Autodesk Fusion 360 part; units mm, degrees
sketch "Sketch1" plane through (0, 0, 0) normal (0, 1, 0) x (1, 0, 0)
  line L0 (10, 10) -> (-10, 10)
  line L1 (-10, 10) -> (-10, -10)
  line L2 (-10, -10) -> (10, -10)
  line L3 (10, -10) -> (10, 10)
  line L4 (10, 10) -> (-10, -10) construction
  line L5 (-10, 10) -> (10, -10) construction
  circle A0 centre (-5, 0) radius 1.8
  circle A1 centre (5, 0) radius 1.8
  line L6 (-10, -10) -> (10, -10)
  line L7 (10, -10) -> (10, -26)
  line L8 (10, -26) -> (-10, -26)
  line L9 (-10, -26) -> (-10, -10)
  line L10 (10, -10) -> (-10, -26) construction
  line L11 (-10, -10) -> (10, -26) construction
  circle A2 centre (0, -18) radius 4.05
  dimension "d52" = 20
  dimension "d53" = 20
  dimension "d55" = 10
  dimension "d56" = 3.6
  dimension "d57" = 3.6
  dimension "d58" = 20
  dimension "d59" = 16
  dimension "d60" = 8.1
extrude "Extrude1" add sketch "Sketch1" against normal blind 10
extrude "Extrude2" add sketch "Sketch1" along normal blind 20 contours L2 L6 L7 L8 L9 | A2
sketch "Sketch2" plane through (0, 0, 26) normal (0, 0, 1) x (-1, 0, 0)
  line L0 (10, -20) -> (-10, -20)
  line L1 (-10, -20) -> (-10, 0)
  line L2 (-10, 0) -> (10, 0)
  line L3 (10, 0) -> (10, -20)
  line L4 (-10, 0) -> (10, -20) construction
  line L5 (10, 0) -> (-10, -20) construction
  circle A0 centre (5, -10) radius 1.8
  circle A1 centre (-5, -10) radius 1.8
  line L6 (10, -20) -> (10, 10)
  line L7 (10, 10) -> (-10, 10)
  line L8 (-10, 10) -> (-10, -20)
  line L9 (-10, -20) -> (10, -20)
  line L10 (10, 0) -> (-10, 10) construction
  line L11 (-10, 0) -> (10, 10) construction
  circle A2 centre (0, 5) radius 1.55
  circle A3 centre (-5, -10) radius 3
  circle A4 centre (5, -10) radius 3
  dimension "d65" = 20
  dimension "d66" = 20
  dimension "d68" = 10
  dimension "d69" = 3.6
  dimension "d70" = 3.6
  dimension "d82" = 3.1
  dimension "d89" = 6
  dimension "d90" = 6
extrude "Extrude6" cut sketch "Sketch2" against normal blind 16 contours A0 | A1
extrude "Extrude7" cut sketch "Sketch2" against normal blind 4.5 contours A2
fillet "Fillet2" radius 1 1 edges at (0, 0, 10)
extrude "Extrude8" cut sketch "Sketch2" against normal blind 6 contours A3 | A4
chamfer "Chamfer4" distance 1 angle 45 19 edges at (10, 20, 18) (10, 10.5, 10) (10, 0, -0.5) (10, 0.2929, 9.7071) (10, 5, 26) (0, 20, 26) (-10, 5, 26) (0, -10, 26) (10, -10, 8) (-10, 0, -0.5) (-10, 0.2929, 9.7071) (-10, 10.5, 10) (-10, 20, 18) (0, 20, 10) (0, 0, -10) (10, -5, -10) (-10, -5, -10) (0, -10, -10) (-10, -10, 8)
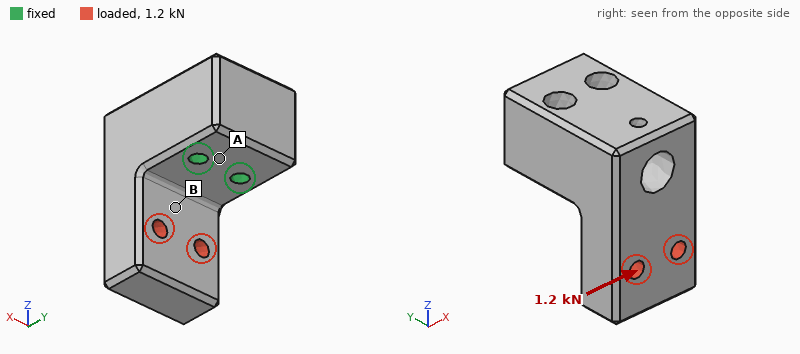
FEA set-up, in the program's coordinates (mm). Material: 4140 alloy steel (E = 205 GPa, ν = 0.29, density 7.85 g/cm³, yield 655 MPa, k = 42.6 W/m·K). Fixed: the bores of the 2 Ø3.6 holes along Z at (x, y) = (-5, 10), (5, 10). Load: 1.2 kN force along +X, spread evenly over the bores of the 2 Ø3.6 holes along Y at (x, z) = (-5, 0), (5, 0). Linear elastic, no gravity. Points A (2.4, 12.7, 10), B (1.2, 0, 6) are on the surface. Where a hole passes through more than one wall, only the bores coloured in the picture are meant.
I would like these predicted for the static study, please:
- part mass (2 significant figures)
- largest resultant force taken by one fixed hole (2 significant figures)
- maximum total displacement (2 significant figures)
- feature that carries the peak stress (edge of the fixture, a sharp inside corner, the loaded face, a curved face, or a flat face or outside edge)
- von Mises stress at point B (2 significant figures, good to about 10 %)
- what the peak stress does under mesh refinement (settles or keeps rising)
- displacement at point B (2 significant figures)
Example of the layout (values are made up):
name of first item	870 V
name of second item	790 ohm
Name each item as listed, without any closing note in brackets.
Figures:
part mass	95 g
largest resultant force taken by one fixed hole	1.8 kN
maximum total displacement	13 µm
feature that carries the peak stress	edge of the fixture
von Mises stress at point B	19 MPa
what the peak stress does under mesh refinement	keeps rising
displacement at point B	5.1 µm
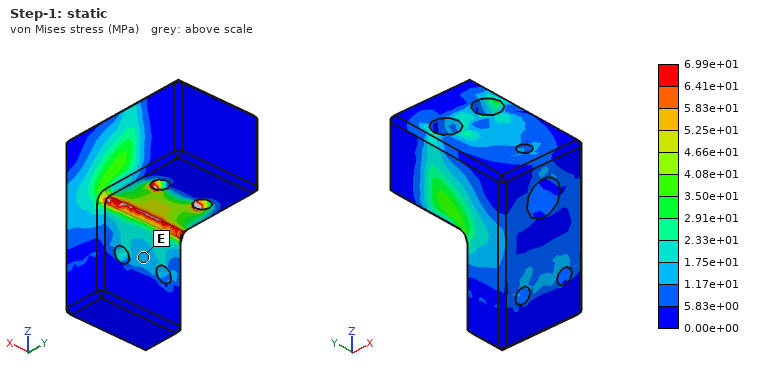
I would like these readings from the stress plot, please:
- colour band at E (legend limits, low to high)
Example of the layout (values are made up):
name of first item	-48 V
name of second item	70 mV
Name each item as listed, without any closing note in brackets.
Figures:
colour band at E	1.17e+01 to 1.75e+01 MPa
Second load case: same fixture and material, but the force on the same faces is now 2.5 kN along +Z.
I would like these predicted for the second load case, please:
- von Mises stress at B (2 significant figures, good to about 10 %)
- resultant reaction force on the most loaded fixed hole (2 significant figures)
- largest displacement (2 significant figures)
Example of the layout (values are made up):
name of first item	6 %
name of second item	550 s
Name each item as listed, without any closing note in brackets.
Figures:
von Mises stress at B	14 MPa
resultant reaction force on the most loaded fixed hole	1.3 kN
largest displacement	17 µm
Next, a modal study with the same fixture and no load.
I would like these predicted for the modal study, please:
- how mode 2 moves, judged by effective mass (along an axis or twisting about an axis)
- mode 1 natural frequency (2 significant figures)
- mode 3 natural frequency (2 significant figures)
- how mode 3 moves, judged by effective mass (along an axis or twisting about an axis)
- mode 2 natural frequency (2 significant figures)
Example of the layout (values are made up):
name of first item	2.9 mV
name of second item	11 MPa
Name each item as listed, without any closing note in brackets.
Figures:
how mode 2 moves, judged by effective mass	along X
mode 1 natural frequency	8000 Hz
mode 3 natural frequency	18 kHz
how mode 3 moves, judged by effective mass	along Z
mode 2 natural frequency	10 kHz
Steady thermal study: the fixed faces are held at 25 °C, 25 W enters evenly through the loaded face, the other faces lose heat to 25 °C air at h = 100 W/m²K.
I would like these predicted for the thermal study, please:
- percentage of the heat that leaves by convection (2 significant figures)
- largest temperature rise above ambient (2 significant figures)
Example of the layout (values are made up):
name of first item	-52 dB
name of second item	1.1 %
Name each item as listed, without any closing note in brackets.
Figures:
percentage of the heat that leaves by convection	34 %
largest temperature rise above ambient	57 K
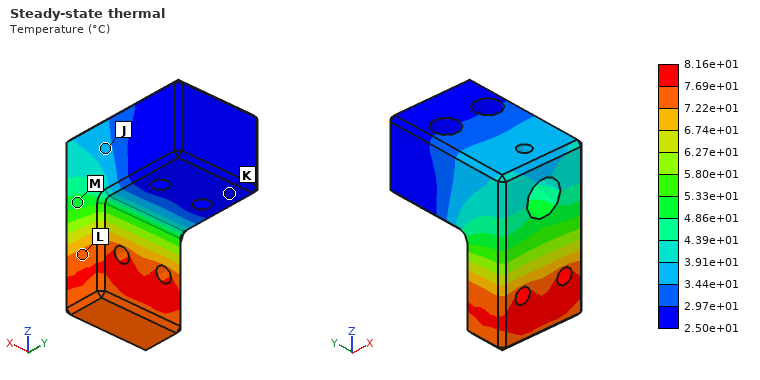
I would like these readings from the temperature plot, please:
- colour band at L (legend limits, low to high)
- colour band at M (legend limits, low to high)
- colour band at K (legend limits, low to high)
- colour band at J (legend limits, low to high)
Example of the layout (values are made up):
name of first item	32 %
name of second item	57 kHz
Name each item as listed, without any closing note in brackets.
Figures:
colour band at L	7.22e+01 to 7.69e+01 °C
colour band at M	4.86e+01 to 5.33e+01 °C
colour band at K	2.50e+01 to 2.97e+01 °C
colour band at J	3.44e+01 to 3.91e+01 °C
